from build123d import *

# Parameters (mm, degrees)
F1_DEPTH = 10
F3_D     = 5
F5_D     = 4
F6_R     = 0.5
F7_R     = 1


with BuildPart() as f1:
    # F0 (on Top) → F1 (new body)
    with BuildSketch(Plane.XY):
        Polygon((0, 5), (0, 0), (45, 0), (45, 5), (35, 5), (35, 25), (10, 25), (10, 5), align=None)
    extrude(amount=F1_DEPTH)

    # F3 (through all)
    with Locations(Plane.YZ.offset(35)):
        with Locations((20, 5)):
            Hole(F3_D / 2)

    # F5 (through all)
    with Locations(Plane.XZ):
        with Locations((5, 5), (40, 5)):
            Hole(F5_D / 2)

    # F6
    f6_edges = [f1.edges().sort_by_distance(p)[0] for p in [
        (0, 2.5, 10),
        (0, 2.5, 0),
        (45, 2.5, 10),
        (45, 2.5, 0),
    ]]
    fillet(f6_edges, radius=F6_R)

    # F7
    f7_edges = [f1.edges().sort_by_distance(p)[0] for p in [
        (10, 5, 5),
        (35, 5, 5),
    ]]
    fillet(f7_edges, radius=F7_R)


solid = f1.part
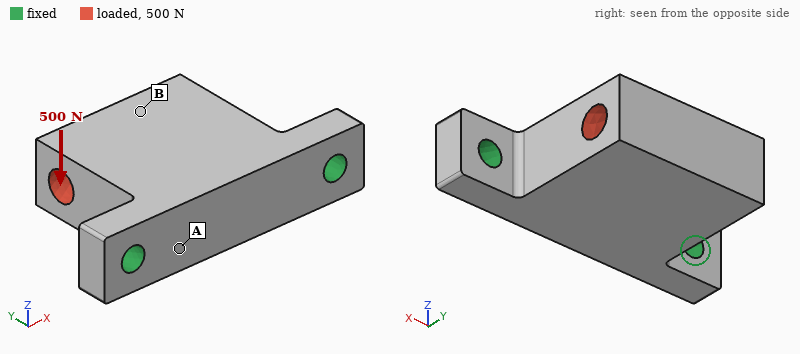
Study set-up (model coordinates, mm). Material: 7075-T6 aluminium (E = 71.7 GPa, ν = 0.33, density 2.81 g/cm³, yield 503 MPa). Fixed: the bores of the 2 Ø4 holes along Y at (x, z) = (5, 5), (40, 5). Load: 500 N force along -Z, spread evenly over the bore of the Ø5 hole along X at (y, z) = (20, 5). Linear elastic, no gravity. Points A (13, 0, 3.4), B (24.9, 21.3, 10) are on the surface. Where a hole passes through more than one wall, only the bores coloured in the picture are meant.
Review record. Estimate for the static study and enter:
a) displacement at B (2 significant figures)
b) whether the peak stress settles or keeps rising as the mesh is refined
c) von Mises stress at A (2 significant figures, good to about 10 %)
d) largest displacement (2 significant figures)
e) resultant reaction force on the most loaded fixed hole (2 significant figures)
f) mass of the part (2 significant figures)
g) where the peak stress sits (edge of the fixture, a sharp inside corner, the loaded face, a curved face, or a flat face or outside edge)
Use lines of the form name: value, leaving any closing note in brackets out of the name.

displacement at B: 62 µm
whether the peak stress settles or keeps rising as the mesh is refined: keeps rising
von Mises stress at A: 31 MPa
largest displacement: 73 µm
resultant reaction force on the most loaded fixed hole: 250 N
mass of the part: 19 g
where the peak stress sits: edge of the fixture
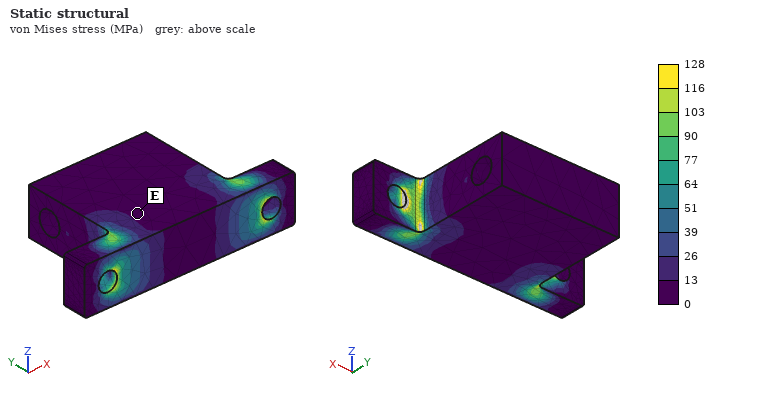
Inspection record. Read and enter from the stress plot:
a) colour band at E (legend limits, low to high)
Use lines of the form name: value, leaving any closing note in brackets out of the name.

colour band at E: 0 to 13 MPa
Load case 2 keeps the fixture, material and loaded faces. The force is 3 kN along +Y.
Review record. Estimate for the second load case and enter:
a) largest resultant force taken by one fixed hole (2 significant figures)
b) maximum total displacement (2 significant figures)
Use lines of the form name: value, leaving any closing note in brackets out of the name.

largest resultant force taken by one fixed hole: 1.7 kN
maximum total displacement: 17 µm
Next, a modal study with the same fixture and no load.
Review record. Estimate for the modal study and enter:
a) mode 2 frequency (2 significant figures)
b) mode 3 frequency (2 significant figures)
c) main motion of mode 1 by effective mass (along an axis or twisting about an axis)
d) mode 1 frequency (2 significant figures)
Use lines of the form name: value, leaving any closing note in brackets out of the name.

mode 2 frequency: 18 kHz
mode 3 frequency: 18 kHz
main motion of mode 1 by effective mass: along Z
mode 1 frequency: 5400 Hz
